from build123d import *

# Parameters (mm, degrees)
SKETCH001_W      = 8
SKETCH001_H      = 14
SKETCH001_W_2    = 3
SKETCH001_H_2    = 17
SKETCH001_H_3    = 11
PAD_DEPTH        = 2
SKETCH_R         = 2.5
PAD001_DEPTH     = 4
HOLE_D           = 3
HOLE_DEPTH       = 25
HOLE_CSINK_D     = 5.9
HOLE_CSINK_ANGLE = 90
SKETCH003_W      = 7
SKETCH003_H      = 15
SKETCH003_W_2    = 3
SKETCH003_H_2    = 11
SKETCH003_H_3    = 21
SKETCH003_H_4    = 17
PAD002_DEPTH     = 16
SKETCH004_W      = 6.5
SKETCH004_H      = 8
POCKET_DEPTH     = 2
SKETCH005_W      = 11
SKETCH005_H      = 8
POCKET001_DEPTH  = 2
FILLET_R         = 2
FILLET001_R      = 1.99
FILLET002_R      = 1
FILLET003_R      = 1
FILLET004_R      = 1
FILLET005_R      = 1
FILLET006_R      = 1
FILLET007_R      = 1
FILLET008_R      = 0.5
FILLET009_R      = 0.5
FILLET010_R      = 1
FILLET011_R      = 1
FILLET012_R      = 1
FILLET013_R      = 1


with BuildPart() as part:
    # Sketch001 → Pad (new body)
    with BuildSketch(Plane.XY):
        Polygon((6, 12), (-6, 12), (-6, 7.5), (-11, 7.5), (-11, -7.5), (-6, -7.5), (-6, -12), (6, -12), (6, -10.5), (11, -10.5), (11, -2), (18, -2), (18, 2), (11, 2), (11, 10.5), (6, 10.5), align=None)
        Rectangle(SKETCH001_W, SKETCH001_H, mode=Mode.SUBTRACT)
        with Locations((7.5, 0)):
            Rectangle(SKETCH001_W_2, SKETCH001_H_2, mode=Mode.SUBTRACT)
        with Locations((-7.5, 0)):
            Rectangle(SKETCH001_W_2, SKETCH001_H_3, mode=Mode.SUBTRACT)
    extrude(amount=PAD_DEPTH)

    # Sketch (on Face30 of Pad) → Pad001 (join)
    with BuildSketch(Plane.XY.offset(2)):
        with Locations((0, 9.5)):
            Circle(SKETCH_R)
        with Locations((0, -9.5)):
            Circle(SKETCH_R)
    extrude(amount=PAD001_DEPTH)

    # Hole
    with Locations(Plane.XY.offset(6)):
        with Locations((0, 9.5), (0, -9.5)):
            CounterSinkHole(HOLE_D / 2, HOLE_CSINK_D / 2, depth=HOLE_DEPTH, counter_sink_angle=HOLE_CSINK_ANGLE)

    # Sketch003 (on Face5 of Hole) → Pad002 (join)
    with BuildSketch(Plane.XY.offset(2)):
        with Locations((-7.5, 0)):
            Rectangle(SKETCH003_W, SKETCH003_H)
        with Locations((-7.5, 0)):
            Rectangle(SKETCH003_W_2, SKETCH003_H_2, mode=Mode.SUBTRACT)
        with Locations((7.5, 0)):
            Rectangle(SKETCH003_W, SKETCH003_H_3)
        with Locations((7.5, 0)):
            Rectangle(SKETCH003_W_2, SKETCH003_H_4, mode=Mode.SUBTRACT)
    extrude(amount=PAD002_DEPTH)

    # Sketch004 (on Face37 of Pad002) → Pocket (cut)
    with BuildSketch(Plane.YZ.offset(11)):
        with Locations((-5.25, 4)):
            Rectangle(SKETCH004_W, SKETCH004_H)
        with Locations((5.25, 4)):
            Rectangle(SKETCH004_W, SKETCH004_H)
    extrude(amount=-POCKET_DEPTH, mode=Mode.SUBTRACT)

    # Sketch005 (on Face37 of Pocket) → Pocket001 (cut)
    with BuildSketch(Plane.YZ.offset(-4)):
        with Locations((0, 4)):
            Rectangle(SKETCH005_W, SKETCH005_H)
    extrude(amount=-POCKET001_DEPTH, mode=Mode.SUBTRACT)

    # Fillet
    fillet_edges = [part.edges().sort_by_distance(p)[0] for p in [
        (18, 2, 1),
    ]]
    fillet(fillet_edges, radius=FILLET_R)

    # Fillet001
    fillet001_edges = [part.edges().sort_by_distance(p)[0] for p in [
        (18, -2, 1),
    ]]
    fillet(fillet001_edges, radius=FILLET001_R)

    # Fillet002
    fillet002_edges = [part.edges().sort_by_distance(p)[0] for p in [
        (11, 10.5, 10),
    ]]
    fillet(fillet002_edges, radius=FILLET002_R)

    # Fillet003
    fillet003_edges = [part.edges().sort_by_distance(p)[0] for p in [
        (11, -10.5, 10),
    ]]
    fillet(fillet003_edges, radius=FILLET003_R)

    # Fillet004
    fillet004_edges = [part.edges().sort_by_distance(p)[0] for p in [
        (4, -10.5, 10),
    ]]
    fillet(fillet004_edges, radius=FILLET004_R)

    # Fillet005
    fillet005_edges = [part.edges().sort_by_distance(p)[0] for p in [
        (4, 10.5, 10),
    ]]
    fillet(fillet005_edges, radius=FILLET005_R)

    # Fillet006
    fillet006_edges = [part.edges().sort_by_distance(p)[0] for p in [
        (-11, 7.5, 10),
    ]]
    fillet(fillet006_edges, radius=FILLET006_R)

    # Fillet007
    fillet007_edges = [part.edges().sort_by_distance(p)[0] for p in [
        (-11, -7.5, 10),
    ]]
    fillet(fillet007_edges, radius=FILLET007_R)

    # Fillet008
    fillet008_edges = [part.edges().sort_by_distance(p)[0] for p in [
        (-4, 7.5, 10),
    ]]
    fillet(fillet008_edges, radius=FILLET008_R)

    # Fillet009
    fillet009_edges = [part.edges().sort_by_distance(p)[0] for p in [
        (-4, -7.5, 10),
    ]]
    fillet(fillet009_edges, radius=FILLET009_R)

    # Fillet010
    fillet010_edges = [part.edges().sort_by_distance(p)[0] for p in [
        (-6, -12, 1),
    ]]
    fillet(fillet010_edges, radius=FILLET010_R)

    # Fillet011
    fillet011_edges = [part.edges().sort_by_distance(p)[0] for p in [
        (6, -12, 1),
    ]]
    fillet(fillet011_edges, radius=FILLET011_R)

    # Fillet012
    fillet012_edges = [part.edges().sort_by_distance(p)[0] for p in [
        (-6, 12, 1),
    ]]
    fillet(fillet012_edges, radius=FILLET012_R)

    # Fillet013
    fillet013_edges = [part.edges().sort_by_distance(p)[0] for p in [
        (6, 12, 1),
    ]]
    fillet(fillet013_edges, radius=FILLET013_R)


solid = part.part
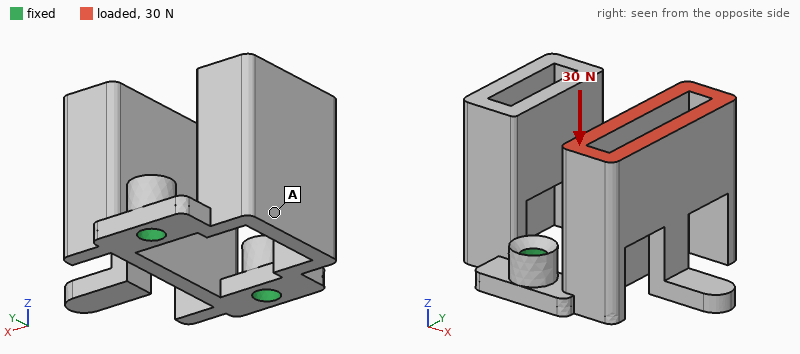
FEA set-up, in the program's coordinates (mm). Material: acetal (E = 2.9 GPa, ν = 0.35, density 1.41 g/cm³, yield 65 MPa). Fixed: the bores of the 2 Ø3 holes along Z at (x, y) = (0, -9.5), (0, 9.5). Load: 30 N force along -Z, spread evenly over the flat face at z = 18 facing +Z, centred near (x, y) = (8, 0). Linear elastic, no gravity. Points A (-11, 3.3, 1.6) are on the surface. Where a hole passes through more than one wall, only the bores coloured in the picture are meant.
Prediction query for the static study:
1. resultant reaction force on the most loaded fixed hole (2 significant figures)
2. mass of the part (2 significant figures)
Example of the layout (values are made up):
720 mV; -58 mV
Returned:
15 N; 4.1 g
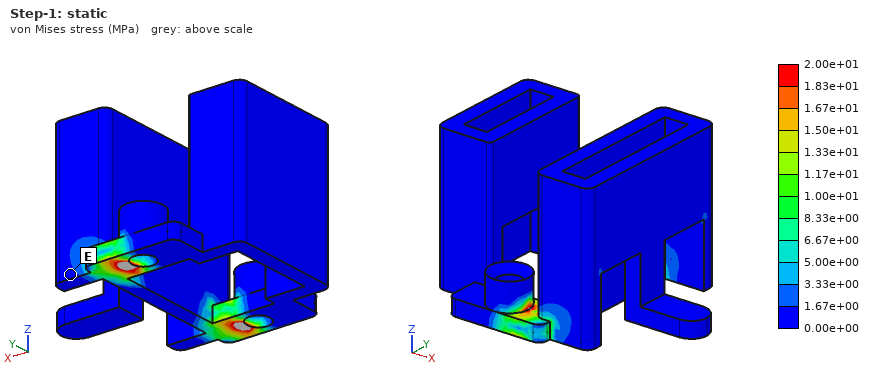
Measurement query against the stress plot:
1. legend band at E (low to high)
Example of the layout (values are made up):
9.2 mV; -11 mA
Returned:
0.00e+00 to 1.67e+00 MPa
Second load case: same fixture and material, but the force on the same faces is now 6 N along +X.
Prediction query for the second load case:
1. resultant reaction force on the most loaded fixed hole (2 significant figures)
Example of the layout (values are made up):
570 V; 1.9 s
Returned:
3.2 N
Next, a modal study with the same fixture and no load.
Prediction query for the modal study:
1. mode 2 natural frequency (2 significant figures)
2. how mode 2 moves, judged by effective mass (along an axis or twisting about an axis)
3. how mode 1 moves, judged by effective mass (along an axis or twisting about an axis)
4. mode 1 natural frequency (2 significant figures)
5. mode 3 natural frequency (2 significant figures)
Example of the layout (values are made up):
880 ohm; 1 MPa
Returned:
680 Hz; along X; along X; 590 Hz; 1800 Hz
